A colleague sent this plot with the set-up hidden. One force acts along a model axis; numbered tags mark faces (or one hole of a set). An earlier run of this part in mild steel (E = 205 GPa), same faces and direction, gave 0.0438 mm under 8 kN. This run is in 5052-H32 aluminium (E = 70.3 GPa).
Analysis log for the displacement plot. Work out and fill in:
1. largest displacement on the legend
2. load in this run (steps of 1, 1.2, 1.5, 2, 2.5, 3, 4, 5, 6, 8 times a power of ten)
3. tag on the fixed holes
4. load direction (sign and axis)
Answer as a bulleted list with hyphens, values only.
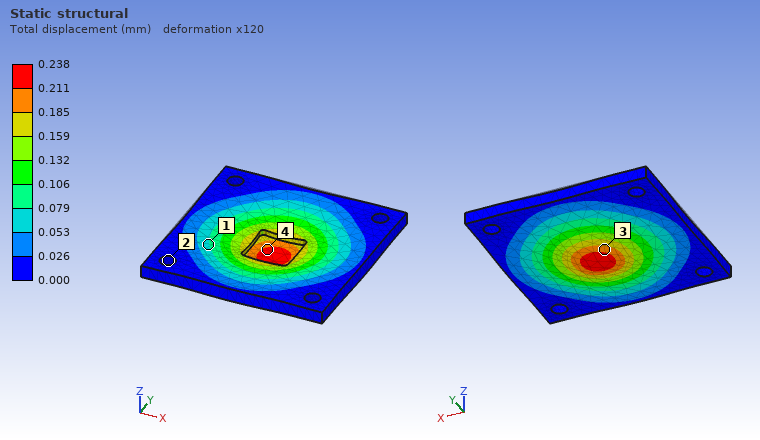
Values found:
- 0.238 mm
- 15 kN
- 2
- -Z
